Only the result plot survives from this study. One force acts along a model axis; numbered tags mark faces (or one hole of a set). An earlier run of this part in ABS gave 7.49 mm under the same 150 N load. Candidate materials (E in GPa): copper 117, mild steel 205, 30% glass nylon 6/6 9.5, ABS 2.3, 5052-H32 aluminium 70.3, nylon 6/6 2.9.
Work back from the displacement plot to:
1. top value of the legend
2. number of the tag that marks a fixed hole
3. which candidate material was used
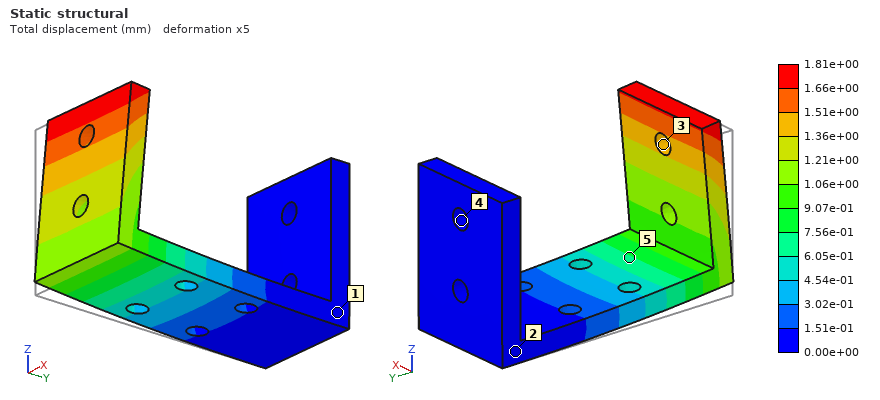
1.81e+00 mm
4
30% glass nylon 6/6
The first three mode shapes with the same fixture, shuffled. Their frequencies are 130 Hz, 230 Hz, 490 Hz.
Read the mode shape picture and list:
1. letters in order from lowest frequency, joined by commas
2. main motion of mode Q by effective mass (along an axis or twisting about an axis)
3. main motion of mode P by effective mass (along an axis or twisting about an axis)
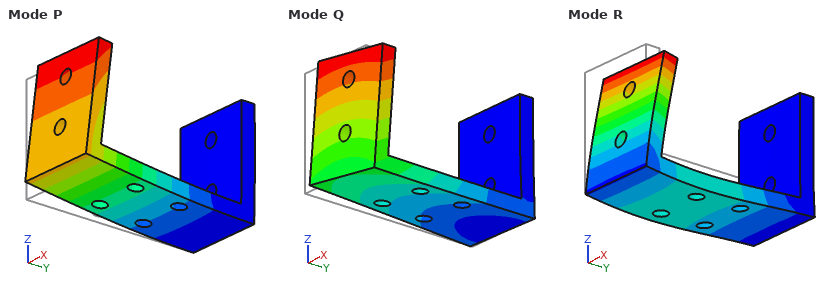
P, Q, R
along X
along Z
